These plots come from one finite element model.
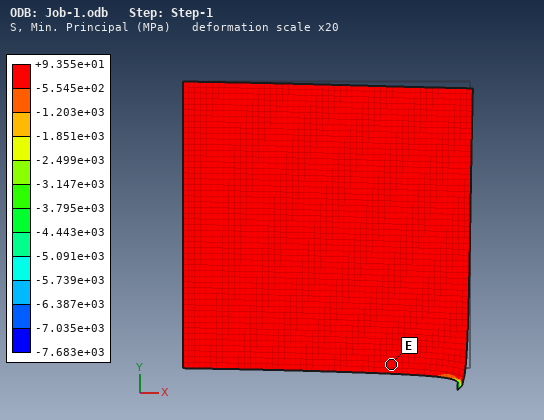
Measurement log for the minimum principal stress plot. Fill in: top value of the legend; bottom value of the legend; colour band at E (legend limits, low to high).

+9.355e+01 MPa
-7.683e+03 MPa
-5.545e+02 to +9.355e+01 MPa
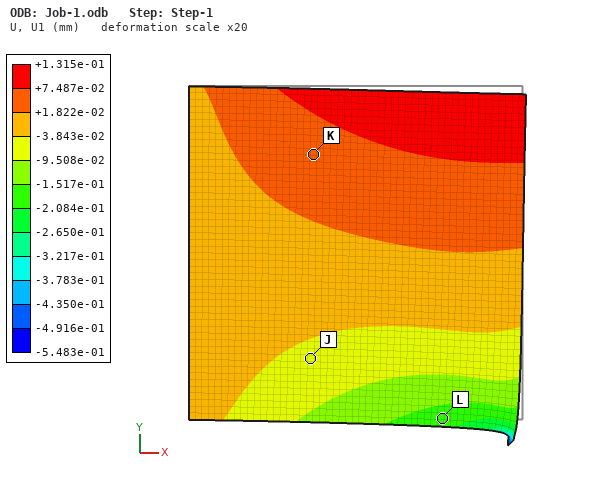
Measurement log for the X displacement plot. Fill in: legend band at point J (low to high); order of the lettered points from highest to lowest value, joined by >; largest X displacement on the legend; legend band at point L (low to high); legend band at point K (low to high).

-9.508e-02 to -3.843e-02 mm
K > J > L
+1.315e-01 mm
-2.084e-01 to -1.517e-01 mm
+1.822e-02 to +7.487e-02 mm
